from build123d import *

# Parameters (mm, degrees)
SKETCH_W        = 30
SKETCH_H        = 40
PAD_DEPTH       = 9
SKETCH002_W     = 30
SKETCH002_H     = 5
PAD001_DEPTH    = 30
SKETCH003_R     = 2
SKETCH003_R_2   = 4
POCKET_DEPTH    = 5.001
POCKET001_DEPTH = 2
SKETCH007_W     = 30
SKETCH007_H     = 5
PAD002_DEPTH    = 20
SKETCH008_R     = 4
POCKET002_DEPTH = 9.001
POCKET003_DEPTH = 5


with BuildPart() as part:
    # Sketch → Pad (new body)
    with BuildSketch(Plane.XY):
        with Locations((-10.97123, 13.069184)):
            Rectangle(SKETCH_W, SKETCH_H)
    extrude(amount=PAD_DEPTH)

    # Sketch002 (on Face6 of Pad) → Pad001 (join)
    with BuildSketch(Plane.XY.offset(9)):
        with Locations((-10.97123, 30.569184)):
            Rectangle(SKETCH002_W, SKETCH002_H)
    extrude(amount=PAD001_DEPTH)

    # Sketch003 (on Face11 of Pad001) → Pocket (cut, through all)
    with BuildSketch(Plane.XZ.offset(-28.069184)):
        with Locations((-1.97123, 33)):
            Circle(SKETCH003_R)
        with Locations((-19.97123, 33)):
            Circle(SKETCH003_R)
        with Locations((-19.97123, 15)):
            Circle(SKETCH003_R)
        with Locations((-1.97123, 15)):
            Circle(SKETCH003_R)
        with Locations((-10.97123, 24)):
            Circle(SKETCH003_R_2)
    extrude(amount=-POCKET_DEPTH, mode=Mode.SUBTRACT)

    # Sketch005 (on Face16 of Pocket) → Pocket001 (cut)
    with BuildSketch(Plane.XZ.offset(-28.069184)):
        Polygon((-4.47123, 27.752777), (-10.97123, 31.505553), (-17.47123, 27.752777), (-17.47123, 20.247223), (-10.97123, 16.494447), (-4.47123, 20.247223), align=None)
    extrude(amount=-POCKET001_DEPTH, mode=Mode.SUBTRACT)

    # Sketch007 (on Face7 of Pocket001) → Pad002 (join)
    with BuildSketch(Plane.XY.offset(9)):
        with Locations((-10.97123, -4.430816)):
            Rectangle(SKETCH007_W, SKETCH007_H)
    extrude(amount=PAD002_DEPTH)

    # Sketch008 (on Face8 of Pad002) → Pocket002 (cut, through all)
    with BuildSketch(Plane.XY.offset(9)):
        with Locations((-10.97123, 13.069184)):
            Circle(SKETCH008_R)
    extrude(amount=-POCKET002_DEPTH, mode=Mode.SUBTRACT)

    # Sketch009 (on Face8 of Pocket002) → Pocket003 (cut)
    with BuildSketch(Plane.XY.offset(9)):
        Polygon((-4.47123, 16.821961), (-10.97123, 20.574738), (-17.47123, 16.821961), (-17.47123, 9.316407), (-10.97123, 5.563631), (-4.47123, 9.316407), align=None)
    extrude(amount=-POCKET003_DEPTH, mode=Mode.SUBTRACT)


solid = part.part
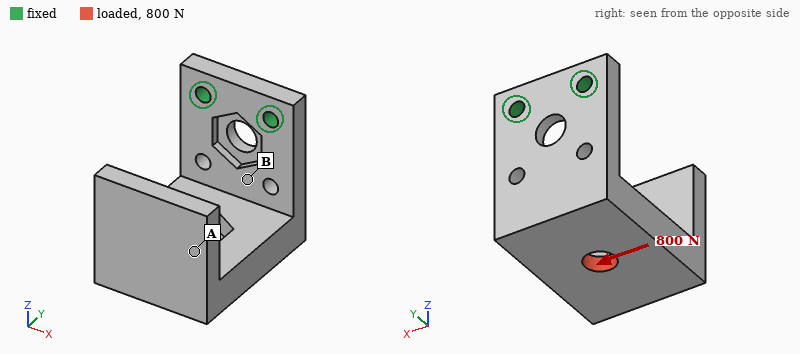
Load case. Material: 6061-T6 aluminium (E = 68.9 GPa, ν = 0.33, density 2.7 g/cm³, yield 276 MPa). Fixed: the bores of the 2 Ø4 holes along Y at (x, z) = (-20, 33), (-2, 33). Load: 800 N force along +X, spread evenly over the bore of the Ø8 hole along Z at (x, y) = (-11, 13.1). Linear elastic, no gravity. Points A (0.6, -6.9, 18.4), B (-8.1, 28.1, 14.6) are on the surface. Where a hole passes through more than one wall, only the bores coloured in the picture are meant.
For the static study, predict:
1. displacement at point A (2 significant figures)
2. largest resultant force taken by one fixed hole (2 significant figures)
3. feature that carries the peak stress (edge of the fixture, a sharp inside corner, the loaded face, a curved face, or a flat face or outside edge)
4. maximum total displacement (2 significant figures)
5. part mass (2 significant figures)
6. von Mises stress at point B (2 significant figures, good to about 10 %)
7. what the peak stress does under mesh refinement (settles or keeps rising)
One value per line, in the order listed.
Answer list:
0.37 mm
1.3 kN
edge of the fixture
0.38 mm
45 g
100 MPa
keeps rising
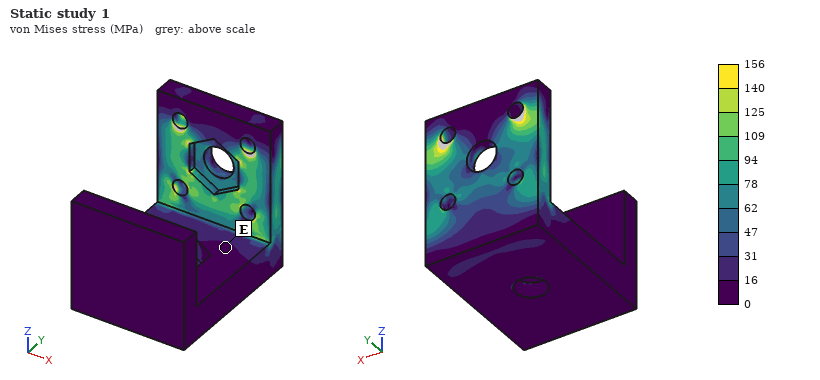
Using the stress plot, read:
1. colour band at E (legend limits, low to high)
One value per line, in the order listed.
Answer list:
0 to 16 MPa
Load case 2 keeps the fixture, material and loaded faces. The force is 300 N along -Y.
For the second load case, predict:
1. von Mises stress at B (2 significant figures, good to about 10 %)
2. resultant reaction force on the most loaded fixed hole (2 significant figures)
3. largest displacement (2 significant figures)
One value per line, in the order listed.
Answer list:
23 MPa
160 N
0.39 mm
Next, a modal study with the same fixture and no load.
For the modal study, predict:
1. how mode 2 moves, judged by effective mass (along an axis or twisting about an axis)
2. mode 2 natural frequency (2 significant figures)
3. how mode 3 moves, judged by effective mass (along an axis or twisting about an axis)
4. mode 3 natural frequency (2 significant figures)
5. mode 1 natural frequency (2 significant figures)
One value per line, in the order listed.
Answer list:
along X
1200 Hz
along Y
2600 Hz
710 Hz
